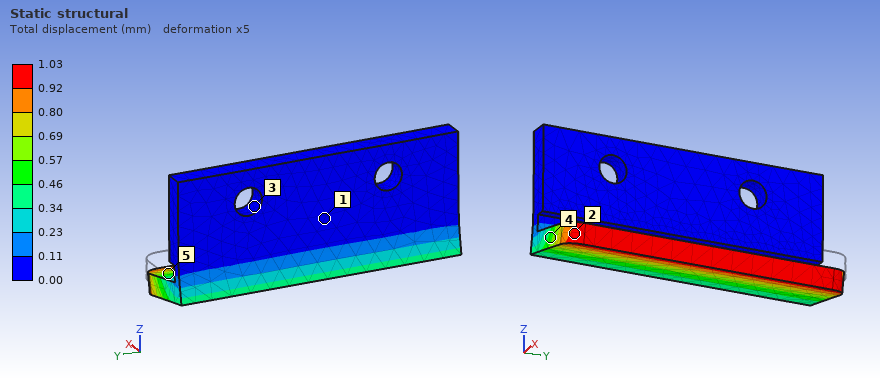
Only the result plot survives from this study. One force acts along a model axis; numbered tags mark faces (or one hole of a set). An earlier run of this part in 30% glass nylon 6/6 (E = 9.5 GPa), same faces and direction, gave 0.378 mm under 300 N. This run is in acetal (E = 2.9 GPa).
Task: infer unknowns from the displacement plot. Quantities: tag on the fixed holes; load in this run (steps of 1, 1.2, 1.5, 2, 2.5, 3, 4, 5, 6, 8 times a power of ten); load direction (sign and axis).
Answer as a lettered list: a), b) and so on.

a) 3
b) 250 N
c) -Z
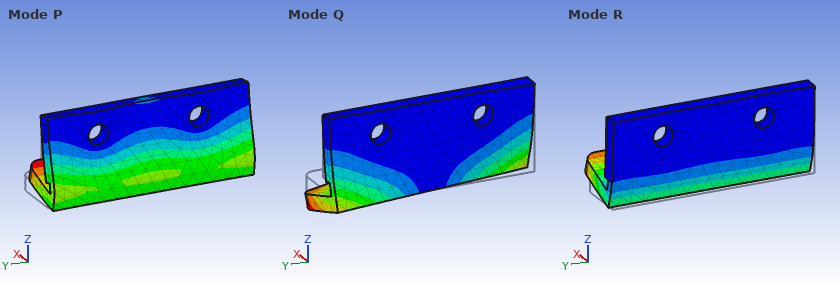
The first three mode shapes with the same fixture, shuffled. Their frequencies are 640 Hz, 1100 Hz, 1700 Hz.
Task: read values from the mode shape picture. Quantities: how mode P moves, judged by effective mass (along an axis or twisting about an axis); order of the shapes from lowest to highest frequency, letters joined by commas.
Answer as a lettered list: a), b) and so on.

a) along X
b) R, Q, P
